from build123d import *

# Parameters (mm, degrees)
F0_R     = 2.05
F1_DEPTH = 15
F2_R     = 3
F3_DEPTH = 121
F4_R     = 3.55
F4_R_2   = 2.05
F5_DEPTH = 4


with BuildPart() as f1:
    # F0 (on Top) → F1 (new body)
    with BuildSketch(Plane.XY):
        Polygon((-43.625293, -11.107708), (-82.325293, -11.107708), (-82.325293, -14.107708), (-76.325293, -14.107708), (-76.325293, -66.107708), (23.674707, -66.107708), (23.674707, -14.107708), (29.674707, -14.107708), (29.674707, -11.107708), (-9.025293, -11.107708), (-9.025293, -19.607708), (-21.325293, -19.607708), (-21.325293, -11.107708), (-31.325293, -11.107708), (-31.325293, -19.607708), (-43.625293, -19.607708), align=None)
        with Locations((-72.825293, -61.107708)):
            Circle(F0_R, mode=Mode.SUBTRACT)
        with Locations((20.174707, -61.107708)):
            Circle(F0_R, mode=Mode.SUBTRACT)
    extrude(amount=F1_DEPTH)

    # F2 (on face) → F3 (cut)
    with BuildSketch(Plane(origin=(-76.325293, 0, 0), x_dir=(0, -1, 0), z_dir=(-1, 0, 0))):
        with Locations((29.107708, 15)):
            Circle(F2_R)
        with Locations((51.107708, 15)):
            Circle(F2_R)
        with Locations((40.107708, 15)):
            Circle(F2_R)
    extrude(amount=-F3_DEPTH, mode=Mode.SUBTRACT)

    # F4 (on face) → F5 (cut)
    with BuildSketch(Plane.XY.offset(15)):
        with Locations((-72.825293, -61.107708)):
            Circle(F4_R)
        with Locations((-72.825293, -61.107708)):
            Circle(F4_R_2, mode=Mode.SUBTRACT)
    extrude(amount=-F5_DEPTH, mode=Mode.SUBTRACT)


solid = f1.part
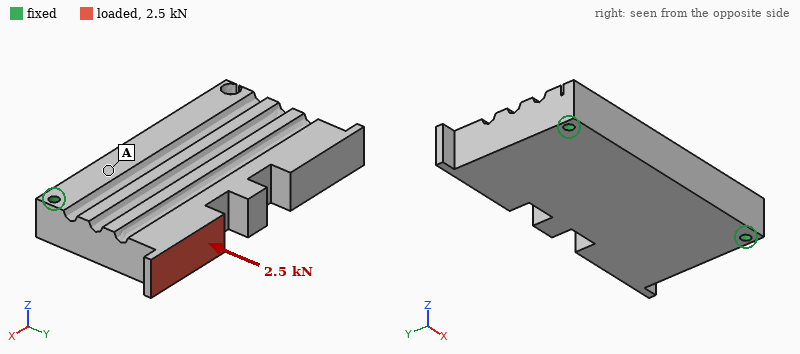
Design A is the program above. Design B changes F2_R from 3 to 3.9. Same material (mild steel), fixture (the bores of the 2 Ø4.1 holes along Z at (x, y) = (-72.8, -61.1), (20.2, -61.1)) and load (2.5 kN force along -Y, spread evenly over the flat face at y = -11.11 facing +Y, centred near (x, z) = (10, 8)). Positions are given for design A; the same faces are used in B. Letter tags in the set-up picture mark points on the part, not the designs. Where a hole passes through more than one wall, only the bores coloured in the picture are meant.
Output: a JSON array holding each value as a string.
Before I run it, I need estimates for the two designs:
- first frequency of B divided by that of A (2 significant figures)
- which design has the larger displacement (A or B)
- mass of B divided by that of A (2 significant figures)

["0.96", "B", "0.96"]
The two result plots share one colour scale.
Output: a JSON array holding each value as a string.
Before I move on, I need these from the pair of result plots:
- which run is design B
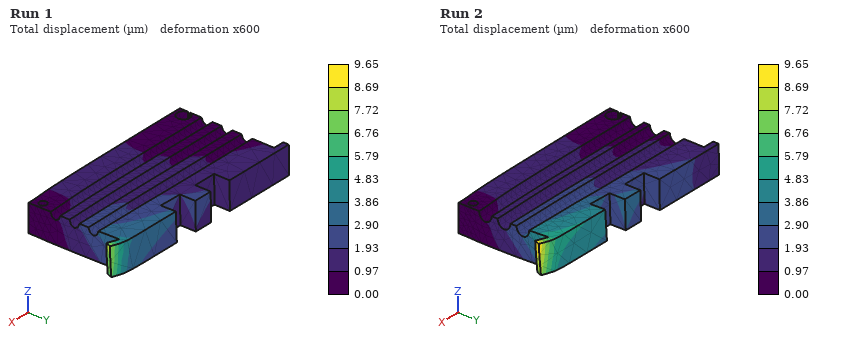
["Run 2"]
